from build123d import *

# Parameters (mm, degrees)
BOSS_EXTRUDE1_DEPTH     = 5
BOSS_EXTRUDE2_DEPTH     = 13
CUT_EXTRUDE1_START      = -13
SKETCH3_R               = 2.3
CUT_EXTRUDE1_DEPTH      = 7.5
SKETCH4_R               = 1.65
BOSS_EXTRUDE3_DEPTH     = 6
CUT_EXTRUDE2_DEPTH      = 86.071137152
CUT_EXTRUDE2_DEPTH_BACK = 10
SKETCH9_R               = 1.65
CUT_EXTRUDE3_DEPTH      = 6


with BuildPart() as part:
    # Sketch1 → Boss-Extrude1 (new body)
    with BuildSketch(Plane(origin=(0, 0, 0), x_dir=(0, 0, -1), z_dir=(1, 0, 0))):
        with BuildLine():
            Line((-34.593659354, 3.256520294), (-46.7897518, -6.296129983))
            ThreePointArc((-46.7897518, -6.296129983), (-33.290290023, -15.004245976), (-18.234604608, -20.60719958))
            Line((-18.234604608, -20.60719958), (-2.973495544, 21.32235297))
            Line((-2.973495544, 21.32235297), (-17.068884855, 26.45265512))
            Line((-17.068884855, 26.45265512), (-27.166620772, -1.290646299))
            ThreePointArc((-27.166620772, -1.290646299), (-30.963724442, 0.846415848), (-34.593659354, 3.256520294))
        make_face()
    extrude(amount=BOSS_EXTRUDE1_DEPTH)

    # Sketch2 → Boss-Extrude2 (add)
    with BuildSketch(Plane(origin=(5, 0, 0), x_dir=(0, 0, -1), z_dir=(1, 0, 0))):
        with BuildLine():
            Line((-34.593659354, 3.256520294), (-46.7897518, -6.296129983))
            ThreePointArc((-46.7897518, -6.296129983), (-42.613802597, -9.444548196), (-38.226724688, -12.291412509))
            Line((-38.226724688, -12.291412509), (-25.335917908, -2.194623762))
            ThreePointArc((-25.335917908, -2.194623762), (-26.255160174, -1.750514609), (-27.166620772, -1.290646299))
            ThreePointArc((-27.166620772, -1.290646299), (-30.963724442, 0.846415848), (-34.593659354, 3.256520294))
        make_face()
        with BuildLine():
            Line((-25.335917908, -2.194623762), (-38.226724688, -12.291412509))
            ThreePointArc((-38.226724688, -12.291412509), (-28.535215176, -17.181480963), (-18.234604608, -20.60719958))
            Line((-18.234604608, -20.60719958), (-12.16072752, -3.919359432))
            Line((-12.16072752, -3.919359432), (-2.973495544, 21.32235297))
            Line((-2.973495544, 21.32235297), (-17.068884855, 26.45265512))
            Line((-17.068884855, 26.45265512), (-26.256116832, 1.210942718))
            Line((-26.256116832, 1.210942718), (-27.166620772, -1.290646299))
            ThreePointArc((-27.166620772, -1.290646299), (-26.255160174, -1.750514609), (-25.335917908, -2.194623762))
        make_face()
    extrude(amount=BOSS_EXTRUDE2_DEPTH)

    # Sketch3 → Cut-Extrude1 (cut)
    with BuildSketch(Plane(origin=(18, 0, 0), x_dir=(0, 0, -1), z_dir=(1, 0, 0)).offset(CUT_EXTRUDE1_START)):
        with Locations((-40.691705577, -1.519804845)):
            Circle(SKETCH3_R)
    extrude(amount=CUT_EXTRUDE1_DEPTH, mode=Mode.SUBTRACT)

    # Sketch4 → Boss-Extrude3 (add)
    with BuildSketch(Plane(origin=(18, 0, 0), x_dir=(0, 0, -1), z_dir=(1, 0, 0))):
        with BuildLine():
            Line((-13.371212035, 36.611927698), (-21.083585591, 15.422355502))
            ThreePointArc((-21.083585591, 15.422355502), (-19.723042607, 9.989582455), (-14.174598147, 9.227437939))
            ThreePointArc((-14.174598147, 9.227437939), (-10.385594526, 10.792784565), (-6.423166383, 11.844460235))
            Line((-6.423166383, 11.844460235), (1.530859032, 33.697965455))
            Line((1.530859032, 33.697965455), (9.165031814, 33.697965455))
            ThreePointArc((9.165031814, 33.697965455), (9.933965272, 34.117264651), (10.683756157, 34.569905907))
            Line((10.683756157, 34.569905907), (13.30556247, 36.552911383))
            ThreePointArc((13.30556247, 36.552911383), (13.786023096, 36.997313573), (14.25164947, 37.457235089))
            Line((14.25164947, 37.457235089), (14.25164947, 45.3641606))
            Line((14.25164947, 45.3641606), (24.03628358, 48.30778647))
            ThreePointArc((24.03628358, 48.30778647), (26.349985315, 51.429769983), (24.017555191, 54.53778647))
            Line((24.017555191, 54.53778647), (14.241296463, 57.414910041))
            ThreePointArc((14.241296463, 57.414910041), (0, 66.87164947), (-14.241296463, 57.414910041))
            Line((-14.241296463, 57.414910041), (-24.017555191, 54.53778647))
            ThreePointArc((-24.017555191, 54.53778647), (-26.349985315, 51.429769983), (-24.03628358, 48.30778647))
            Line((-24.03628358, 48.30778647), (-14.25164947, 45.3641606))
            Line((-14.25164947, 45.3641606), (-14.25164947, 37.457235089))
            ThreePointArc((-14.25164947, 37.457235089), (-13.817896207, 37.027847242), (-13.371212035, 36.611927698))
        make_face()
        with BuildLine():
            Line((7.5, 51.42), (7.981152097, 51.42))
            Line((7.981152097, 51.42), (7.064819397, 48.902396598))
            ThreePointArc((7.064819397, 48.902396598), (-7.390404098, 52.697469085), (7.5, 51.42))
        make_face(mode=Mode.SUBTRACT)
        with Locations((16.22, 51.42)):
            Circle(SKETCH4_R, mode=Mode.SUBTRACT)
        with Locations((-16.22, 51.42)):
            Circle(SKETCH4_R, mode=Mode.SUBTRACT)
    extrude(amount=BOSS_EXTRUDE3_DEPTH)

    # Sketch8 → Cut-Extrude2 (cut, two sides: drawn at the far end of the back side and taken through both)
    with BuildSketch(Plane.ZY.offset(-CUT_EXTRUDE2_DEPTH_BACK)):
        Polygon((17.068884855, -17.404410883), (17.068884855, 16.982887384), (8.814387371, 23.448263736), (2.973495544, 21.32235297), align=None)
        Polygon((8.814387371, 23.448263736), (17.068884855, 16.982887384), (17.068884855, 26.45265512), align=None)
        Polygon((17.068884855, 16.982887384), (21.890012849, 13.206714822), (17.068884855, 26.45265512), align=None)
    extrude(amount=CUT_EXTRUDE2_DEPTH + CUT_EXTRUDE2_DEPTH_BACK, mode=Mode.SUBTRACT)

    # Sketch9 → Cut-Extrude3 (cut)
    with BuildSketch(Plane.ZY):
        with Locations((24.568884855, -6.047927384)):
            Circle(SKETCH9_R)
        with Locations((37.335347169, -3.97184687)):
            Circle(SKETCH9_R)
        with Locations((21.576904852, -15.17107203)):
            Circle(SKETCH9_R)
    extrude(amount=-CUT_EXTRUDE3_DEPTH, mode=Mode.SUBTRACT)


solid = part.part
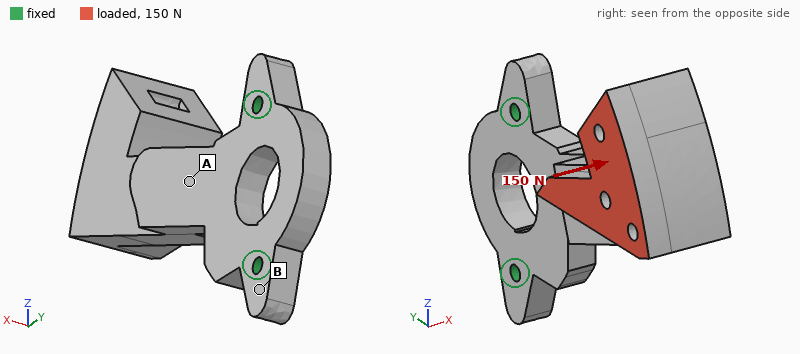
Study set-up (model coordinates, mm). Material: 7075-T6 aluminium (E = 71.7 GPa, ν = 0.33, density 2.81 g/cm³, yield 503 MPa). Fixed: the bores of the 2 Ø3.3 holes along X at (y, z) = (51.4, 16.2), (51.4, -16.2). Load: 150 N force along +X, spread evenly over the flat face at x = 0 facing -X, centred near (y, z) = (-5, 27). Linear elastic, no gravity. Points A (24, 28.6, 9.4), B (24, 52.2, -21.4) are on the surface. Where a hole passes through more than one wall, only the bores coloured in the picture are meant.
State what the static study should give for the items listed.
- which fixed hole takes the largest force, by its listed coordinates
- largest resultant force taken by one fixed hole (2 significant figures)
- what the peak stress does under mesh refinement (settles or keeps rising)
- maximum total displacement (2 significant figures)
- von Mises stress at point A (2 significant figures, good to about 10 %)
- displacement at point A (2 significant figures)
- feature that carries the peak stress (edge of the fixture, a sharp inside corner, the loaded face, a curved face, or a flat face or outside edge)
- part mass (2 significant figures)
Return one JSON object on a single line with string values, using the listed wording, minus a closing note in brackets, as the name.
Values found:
{"which fixed hole takes the largest force, by its listed coordinates": "(51.4, 16.2)", "largest resultant force taken by one fixed hole": "220 N", "what the peak stress does under mesh refinement": "keeps rising", "maximum total displacement": "0.69 mm", "von Mises stress at point A": "60 MPa", "displacement at point A": "0.12 mm", "feature that carries the peak stress": "edge of the fixture", "part mass": "55 g"}
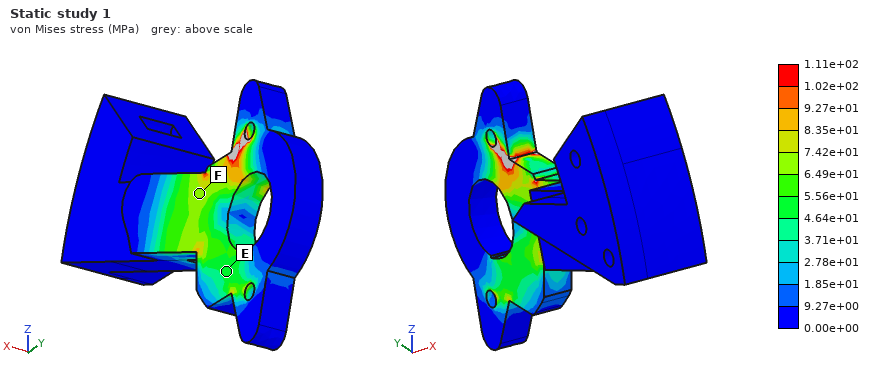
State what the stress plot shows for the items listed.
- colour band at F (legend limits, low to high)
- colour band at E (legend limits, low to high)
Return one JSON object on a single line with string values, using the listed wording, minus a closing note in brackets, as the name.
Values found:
{"colour band at F": "6.49e+01 to 7.42e+01 MPa", "colour band at E": "4.64e+01 to 5.56e+01 MPa"}
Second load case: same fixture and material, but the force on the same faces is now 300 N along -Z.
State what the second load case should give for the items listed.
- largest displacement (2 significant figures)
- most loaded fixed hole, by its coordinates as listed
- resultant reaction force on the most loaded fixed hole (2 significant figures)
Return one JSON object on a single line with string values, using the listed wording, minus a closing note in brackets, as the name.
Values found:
{"largest displacement": "0.38 mm", "most loaded fixed hole, by its coordinates as listed": "(51.4, -16.2)", "resultant reaction force on the most loaded fixed hole": "720 N"}
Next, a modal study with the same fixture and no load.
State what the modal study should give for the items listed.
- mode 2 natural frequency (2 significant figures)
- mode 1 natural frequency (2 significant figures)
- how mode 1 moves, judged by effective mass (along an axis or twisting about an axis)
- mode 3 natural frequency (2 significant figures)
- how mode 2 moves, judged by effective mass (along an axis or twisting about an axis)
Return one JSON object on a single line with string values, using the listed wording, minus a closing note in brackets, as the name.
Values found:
{"mode 2 natural frequency": "1200 Hz", "mode 1 natural frequency": "470 Hz", "how mode 1 moves, judged by effective mass": "along X", "mode 3 natural frequency": "3000 Hz", "how mode 2 moves, judged by effective mass": "along Z"}
